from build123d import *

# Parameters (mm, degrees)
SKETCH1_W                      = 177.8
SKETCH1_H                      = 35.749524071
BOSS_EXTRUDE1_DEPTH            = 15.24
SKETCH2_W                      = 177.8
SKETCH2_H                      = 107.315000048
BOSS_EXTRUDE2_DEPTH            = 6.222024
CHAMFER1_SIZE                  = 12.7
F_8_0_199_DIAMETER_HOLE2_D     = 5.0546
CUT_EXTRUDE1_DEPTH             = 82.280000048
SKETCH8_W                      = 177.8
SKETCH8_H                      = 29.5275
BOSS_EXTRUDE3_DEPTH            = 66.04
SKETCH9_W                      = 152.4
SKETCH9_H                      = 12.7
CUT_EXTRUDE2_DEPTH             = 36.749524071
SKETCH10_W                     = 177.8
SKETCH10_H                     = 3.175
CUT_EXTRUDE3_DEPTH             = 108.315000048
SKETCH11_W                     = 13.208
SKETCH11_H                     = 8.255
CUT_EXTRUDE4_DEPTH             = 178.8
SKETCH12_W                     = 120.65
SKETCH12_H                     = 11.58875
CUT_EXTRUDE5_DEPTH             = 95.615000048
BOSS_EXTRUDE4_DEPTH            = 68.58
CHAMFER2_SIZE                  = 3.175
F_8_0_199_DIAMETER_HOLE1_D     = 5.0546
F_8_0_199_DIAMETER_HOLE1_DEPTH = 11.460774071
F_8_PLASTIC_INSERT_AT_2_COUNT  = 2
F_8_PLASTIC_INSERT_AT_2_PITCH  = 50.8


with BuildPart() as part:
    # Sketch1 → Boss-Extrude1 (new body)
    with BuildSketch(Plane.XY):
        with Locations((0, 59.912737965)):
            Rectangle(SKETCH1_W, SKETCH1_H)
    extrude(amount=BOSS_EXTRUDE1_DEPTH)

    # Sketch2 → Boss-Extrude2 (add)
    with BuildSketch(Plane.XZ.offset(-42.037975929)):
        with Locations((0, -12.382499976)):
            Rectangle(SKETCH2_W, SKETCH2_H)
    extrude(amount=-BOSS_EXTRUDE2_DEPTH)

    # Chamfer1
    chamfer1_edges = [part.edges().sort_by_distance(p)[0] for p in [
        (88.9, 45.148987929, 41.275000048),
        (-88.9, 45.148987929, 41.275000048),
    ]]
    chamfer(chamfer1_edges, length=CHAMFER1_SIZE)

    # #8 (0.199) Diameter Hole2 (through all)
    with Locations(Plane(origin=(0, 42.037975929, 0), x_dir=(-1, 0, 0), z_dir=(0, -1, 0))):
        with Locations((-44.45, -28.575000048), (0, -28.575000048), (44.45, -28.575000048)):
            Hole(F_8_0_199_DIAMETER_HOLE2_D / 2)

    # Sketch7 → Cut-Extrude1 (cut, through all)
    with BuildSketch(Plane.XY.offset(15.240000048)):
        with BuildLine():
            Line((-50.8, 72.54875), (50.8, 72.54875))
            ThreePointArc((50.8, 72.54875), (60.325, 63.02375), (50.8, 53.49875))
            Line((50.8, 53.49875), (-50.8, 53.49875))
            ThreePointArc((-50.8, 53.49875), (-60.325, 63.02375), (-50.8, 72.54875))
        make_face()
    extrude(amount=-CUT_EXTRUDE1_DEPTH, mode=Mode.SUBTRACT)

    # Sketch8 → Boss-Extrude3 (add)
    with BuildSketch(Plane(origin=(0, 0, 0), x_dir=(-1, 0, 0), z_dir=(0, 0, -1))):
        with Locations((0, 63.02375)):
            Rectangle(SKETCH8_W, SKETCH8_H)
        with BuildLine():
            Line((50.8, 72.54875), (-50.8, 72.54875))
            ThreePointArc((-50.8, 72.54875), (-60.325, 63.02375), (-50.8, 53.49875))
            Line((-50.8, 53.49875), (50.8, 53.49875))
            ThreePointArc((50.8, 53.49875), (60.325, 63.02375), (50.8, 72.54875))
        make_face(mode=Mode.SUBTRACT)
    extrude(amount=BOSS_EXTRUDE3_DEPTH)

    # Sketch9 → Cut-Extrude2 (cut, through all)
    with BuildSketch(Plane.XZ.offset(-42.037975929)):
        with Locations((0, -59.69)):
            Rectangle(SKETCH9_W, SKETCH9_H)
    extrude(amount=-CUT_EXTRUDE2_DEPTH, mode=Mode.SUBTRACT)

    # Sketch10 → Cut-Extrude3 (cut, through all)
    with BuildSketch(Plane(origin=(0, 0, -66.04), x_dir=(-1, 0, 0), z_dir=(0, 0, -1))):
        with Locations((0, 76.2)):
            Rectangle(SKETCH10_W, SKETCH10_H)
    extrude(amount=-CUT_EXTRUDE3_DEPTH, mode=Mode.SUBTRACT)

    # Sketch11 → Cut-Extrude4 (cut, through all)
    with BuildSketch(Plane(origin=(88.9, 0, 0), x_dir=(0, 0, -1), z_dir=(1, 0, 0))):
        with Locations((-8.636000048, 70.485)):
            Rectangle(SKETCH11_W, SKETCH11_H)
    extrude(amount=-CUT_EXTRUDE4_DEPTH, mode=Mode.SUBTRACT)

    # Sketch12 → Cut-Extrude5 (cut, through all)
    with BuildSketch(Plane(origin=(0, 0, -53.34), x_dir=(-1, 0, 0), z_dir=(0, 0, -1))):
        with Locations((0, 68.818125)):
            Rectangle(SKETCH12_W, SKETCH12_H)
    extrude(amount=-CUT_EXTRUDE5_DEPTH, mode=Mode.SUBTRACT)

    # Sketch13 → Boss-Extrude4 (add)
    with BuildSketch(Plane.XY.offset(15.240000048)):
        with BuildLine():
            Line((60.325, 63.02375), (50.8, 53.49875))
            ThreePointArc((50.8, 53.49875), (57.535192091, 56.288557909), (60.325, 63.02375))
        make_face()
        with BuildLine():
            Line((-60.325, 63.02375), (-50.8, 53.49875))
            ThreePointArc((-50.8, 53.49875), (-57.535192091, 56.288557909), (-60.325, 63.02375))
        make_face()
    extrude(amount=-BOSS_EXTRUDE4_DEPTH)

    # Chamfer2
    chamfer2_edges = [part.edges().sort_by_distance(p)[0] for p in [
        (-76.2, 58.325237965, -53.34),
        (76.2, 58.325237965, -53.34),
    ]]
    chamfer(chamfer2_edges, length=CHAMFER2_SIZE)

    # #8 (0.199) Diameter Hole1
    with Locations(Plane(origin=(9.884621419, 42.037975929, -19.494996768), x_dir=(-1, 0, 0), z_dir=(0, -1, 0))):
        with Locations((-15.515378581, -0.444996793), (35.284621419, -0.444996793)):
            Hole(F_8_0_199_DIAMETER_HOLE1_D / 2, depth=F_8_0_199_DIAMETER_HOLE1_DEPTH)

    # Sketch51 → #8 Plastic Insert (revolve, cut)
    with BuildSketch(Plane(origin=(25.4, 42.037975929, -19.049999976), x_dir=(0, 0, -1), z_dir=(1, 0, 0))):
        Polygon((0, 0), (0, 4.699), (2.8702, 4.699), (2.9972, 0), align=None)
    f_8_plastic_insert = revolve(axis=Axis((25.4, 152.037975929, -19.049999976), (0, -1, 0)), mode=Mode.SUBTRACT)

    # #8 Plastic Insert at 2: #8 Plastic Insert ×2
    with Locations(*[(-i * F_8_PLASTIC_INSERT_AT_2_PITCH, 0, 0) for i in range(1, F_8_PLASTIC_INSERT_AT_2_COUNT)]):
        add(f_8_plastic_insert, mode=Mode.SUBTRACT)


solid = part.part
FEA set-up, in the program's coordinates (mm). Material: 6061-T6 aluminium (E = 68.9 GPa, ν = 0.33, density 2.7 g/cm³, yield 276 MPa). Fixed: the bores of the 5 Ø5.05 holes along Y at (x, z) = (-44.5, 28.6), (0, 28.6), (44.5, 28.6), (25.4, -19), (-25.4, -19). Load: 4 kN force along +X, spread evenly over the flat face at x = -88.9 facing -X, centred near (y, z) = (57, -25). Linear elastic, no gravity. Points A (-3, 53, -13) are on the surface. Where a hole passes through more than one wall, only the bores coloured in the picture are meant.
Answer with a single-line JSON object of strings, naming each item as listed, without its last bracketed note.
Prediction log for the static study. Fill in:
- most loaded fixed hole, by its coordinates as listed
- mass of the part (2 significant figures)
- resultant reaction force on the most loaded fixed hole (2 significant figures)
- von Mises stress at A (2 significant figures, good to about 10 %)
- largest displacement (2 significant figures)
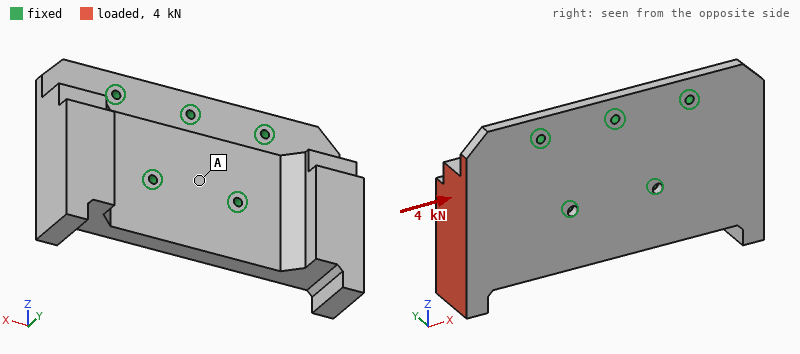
{"most loaded fixed hole, by its coordinates as listed": "(-25.4, -19)", "mass of the part": "700 g", "resultant reaction force on the most loaded fixed hole": "3.1 kN", "von Mises stress at A": "3.2 MPa", "largest displacement": "0.12 mm"}
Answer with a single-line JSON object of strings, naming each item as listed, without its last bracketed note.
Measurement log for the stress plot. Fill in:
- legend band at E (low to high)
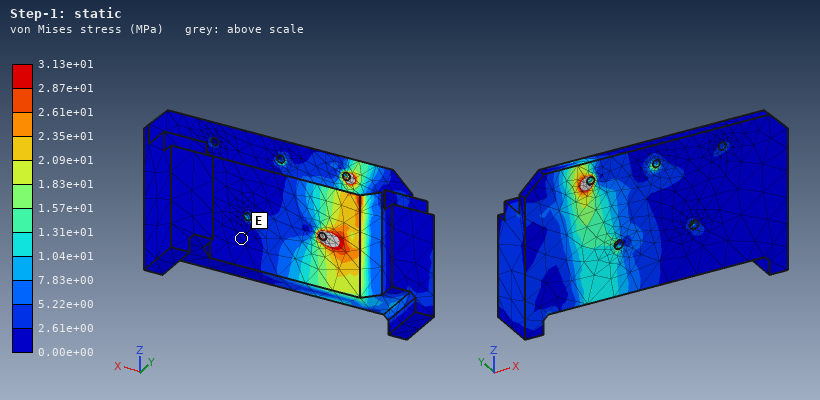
{"legend band at E": "0.00e+00 to 2.61e+00 MPa"}
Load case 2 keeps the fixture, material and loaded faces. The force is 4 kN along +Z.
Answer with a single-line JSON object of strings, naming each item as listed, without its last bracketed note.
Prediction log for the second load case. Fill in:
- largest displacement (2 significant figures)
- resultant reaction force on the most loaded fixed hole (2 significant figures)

{"largest displacement": "90 µm", "resultant reaction force on the most loaded fixed hole": "3.4 kN"}
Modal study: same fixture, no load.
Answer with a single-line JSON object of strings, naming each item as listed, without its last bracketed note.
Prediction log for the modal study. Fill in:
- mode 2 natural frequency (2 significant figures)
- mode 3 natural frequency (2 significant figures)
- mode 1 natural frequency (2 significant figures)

{"mode 2 natural frequency": "1200 Hz", "mode 3 natural frequency": "3300 Hz", "mode 1 natural frequency": "1200 Hz"}
